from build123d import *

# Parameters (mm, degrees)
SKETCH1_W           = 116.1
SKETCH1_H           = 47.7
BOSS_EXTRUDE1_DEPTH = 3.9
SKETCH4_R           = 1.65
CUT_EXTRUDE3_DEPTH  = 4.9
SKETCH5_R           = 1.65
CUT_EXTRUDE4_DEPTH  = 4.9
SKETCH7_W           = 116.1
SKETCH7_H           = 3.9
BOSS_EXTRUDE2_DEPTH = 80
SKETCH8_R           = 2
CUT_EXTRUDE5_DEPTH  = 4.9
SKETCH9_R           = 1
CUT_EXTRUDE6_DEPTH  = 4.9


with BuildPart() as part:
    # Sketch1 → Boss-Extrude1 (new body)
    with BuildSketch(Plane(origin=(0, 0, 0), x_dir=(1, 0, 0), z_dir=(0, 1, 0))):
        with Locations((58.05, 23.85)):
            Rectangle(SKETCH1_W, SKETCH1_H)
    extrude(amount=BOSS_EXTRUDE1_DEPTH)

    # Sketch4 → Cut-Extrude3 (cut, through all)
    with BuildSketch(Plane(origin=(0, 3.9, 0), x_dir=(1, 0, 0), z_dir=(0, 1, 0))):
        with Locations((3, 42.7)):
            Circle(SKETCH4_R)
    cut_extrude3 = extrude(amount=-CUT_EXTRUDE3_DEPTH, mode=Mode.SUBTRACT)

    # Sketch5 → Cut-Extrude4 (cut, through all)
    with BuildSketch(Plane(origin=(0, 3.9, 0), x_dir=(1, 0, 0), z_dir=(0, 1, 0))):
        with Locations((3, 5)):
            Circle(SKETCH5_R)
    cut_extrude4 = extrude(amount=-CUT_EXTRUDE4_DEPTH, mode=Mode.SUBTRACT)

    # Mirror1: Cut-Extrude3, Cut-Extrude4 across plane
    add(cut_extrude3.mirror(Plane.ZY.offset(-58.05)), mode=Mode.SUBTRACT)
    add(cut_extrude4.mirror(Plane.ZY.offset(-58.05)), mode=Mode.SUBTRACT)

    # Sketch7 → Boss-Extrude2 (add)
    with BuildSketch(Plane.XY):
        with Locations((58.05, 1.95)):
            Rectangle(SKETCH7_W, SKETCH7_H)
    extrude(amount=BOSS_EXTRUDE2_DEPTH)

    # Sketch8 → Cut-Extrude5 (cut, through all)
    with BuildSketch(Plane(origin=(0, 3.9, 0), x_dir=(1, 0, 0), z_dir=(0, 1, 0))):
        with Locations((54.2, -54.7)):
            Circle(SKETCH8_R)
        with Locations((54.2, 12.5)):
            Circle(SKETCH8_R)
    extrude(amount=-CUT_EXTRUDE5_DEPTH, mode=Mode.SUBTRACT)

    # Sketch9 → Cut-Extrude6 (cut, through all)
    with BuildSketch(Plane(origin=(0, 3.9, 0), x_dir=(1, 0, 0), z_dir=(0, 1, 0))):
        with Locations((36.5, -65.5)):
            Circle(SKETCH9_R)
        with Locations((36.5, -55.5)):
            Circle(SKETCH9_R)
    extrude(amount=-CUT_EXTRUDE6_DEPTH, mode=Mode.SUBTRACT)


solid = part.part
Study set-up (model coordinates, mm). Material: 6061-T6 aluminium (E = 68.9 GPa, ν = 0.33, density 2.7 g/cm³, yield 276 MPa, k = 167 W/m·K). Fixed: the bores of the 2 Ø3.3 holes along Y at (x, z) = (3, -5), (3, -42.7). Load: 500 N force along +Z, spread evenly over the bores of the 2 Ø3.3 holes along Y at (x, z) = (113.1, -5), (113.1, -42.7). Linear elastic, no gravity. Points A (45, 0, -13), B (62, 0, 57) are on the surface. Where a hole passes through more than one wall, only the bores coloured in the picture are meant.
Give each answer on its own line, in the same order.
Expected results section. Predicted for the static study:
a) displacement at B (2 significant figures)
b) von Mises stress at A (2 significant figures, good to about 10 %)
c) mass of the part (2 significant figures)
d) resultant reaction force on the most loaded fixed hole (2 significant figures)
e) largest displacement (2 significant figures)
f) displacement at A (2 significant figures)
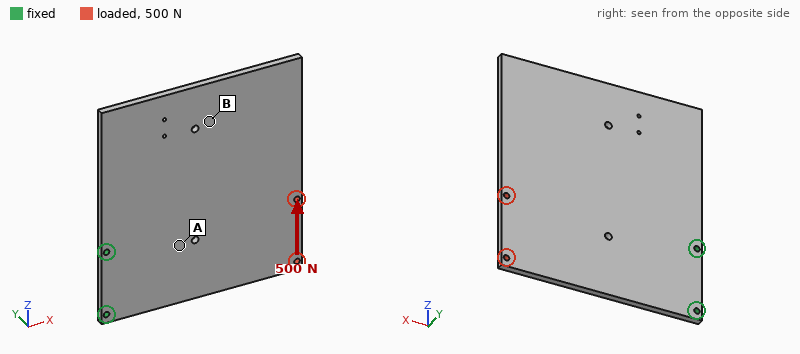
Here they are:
59 µm
7.5 MPa
160 g
1.5 kN
93 µm
23 µm
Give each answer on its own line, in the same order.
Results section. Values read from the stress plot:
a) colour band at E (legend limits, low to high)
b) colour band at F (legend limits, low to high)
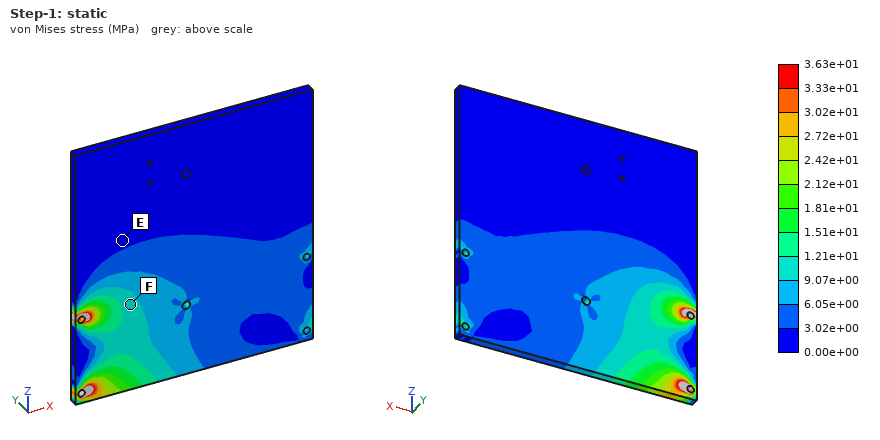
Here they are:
0.00e+00 to 3.02e+00 MPa
9.07e+00 to 1.21e+01 MPa
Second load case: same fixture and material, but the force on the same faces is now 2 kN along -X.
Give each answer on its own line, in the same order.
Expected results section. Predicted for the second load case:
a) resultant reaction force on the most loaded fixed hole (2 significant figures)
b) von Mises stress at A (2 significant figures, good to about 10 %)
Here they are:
1.0 kN
6.4 MPa
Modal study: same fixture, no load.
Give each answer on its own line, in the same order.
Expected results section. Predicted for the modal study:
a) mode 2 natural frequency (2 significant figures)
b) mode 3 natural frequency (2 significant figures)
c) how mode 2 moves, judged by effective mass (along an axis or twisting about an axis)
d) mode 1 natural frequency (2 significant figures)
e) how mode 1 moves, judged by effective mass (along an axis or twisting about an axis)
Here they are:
320 Hz
760 Hz
twisting about X
160 Hz
along Y
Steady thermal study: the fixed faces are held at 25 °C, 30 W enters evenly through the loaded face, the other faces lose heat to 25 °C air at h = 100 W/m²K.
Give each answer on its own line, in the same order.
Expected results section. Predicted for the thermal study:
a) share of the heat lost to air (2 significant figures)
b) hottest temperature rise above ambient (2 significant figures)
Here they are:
85 %
48 K
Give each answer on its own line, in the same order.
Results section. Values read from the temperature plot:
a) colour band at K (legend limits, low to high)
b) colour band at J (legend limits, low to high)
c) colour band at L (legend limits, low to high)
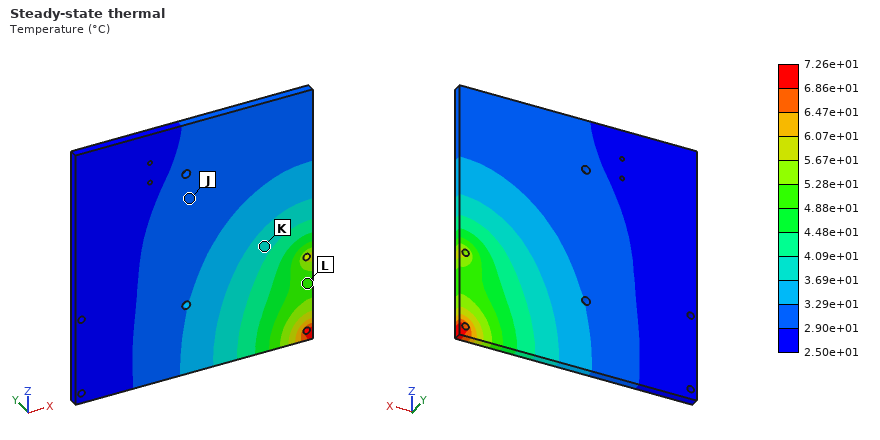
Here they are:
3.69e+01 to 4.09e+01 °C
2.90e+01 to 3.29e+01 °C
4.88e+01 to 5.28e+01 °C
